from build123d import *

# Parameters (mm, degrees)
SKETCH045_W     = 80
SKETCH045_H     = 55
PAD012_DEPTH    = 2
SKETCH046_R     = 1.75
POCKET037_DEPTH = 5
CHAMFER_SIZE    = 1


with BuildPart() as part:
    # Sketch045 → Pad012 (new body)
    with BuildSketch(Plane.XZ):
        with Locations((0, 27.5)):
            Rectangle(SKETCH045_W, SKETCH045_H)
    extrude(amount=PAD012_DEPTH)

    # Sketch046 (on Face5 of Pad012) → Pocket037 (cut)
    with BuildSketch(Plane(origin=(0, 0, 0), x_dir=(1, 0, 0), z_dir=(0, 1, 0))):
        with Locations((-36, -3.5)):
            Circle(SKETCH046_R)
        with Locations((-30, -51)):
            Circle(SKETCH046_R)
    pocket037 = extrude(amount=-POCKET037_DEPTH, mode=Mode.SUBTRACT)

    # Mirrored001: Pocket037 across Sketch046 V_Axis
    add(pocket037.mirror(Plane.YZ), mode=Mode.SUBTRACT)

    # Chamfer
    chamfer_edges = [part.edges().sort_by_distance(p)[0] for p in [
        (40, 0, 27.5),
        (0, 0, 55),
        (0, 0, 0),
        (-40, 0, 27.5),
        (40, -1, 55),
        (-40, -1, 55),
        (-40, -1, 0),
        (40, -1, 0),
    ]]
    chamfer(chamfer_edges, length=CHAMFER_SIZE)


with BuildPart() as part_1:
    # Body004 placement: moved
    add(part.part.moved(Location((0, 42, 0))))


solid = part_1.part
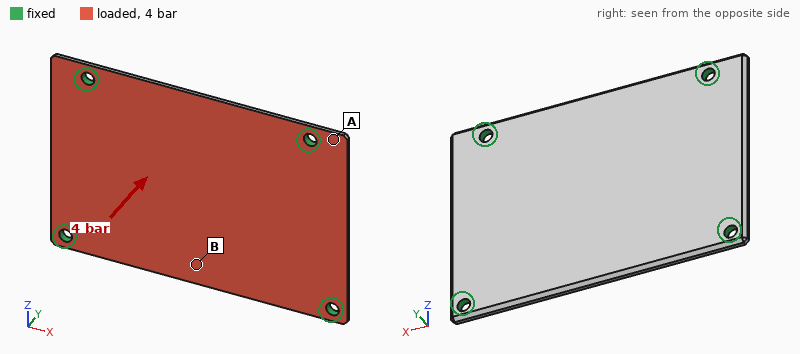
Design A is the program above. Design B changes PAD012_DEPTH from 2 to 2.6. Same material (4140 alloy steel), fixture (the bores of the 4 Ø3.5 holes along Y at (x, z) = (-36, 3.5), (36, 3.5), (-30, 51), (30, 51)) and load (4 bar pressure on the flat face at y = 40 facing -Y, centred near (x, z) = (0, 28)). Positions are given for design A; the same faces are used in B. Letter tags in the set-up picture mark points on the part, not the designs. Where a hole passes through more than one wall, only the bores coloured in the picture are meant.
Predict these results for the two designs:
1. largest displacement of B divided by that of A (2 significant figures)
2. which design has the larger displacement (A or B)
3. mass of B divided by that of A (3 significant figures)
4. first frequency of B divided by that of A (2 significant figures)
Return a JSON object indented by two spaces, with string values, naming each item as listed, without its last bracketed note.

{
  "largest displacement of B divided by that of A": "0.47",
  "which design has the larger displacement": "A",
  "mass of B divided by that of A": "1.30",
  "first frequency of B divided by that of A": "1.3"
}
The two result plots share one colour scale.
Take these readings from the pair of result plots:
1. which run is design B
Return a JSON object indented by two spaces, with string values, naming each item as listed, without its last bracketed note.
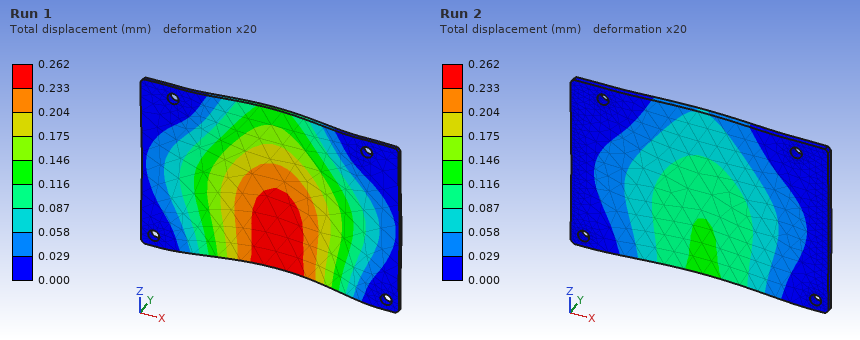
{
  "which run is design B": "Run 2"
}
